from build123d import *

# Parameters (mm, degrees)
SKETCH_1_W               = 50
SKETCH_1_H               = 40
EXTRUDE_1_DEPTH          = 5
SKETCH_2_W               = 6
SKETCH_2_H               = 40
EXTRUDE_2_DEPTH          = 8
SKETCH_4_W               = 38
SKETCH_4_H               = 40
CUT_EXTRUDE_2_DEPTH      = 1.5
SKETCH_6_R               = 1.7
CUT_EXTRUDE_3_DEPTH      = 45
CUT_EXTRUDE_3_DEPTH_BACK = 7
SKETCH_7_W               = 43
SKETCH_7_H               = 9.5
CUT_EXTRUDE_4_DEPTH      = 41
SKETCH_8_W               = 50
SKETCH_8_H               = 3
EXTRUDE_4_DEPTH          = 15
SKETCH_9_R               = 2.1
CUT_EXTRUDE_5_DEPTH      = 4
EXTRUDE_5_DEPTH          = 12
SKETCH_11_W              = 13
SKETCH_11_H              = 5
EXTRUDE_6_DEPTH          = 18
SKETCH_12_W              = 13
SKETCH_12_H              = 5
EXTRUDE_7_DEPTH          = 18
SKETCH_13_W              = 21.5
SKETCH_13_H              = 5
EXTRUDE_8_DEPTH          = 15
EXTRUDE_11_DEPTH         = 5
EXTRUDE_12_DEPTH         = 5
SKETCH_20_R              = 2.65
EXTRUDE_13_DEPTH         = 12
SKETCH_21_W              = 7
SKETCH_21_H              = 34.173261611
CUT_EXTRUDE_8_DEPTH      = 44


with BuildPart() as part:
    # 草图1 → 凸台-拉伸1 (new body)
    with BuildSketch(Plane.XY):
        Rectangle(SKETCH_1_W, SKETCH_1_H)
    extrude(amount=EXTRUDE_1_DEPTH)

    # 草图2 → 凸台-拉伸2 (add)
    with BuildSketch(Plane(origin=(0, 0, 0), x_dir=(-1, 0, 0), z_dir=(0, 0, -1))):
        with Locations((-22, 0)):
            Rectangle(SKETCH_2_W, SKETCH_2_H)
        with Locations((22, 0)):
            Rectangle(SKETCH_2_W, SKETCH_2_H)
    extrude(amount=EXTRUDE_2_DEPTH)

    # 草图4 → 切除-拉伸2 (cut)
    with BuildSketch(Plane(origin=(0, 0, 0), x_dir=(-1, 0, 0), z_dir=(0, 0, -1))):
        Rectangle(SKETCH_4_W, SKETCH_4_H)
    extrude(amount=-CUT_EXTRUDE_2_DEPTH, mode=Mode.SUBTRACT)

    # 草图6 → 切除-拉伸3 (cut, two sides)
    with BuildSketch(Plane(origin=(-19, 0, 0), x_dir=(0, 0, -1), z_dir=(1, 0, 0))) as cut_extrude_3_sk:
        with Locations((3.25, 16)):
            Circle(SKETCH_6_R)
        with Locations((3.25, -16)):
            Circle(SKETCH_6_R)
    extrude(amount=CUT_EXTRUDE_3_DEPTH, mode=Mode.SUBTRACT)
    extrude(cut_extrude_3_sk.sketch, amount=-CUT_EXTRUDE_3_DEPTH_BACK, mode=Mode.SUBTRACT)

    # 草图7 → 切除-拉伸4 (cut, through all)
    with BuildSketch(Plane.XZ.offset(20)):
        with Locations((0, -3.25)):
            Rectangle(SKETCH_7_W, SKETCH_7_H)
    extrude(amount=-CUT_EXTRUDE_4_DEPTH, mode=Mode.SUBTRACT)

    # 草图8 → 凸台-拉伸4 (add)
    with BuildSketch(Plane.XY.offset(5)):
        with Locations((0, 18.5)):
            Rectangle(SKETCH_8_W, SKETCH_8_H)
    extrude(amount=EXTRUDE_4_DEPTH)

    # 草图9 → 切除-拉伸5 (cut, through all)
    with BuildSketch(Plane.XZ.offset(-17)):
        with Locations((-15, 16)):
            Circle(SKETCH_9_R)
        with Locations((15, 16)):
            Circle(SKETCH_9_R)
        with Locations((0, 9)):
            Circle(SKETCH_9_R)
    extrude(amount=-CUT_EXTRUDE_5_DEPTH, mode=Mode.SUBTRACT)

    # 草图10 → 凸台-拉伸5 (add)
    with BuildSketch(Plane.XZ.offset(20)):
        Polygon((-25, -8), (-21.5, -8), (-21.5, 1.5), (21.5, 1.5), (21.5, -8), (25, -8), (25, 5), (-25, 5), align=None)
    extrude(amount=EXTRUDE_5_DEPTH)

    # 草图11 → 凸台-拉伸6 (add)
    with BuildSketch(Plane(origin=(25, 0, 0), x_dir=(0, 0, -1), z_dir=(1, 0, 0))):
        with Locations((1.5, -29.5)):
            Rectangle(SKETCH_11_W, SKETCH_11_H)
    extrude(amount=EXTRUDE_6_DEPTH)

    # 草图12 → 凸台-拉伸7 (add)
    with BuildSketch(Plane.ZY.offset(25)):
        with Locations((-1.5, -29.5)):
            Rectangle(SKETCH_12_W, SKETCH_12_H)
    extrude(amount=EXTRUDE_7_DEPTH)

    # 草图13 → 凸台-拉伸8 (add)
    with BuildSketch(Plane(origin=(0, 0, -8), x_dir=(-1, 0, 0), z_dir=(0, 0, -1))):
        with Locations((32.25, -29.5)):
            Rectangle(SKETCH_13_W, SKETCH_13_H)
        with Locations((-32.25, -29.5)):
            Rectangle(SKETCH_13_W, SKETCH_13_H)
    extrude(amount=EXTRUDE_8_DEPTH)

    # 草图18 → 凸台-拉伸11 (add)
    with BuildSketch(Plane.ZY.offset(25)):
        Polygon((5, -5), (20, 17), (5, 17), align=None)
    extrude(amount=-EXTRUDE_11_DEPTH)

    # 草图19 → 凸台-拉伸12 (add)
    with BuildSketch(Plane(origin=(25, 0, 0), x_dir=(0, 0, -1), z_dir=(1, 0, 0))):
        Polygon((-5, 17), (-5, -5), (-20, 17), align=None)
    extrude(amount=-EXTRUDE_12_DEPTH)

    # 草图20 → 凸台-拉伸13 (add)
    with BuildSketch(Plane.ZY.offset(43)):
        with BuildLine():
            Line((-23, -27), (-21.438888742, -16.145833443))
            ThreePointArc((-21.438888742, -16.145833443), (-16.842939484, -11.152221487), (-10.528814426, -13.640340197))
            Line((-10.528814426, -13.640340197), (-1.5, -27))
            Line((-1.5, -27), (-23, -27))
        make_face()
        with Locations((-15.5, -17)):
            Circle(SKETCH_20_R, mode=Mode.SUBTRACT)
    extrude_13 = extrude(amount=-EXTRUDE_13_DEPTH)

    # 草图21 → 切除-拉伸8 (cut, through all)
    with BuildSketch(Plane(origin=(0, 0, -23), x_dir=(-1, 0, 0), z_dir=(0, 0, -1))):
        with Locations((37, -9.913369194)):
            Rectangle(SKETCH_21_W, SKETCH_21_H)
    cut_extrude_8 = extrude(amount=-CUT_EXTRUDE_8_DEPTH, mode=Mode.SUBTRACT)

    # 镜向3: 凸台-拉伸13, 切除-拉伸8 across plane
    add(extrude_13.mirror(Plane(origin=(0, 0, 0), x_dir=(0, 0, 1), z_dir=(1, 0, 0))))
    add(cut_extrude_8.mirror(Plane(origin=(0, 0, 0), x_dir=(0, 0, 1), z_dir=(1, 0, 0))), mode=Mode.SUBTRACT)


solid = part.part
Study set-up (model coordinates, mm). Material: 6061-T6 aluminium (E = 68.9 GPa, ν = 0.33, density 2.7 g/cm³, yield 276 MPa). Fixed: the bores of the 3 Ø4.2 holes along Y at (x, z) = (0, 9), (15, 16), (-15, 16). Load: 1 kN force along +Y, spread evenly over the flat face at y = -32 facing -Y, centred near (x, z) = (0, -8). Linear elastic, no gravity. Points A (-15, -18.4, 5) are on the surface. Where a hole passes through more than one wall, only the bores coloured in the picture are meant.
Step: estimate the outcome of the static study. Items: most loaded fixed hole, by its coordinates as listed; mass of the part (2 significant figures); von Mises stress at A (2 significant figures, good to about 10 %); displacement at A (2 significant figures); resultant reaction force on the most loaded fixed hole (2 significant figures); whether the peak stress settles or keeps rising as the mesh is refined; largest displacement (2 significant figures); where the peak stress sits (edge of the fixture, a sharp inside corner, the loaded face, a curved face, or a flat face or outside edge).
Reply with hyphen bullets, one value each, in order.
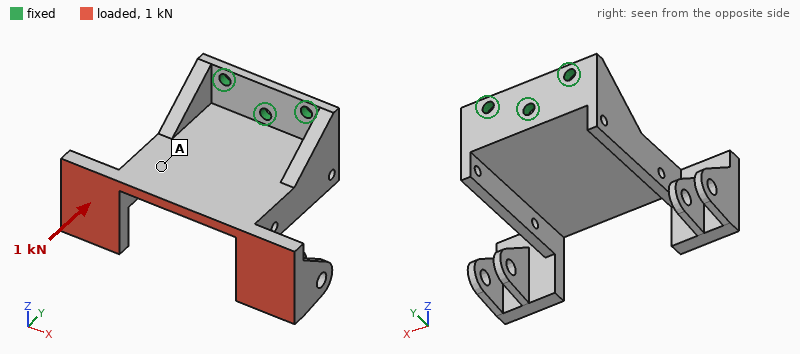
- (0, 9)
- 64 g
- 16 MPa
- 0.18 mm
- 1.7 kN
- keeps rising
- 0.39 mm
- edge of the fixture
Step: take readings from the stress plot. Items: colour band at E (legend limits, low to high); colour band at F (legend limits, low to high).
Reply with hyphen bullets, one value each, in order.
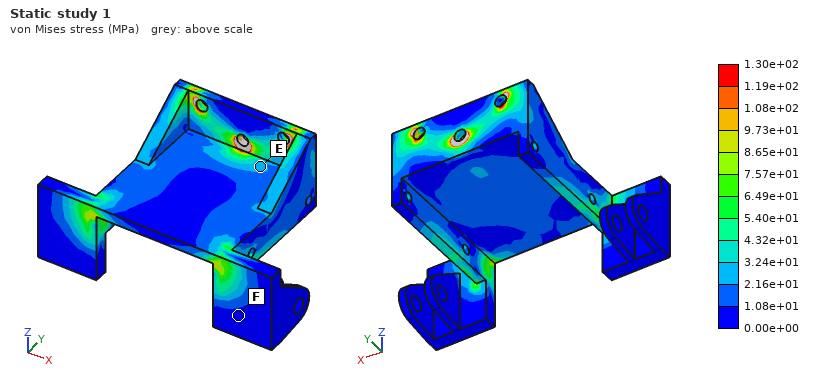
- 2.16e+01 to 3.24e+01 MPa
- 0.00e+00 to 1.08e+01 MPa
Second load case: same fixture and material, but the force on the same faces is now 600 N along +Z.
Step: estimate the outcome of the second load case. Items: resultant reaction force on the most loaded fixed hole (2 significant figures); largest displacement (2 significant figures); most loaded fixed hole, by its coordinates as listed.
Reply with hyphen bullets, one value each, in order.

- 2.1 kN
- 0.65 mm
- (0, 9)
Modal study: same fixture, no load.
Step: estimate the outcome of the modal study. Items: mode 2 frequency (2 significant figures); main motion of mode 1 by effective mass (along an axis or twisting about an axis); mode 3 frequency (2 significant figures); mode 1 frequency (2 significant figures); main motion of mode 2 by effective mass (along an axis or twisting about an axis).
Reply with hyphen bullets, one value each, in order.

- 1000 Hz
- twisting about Y
- 1500 Hz
- 870 Hz
- along Z
